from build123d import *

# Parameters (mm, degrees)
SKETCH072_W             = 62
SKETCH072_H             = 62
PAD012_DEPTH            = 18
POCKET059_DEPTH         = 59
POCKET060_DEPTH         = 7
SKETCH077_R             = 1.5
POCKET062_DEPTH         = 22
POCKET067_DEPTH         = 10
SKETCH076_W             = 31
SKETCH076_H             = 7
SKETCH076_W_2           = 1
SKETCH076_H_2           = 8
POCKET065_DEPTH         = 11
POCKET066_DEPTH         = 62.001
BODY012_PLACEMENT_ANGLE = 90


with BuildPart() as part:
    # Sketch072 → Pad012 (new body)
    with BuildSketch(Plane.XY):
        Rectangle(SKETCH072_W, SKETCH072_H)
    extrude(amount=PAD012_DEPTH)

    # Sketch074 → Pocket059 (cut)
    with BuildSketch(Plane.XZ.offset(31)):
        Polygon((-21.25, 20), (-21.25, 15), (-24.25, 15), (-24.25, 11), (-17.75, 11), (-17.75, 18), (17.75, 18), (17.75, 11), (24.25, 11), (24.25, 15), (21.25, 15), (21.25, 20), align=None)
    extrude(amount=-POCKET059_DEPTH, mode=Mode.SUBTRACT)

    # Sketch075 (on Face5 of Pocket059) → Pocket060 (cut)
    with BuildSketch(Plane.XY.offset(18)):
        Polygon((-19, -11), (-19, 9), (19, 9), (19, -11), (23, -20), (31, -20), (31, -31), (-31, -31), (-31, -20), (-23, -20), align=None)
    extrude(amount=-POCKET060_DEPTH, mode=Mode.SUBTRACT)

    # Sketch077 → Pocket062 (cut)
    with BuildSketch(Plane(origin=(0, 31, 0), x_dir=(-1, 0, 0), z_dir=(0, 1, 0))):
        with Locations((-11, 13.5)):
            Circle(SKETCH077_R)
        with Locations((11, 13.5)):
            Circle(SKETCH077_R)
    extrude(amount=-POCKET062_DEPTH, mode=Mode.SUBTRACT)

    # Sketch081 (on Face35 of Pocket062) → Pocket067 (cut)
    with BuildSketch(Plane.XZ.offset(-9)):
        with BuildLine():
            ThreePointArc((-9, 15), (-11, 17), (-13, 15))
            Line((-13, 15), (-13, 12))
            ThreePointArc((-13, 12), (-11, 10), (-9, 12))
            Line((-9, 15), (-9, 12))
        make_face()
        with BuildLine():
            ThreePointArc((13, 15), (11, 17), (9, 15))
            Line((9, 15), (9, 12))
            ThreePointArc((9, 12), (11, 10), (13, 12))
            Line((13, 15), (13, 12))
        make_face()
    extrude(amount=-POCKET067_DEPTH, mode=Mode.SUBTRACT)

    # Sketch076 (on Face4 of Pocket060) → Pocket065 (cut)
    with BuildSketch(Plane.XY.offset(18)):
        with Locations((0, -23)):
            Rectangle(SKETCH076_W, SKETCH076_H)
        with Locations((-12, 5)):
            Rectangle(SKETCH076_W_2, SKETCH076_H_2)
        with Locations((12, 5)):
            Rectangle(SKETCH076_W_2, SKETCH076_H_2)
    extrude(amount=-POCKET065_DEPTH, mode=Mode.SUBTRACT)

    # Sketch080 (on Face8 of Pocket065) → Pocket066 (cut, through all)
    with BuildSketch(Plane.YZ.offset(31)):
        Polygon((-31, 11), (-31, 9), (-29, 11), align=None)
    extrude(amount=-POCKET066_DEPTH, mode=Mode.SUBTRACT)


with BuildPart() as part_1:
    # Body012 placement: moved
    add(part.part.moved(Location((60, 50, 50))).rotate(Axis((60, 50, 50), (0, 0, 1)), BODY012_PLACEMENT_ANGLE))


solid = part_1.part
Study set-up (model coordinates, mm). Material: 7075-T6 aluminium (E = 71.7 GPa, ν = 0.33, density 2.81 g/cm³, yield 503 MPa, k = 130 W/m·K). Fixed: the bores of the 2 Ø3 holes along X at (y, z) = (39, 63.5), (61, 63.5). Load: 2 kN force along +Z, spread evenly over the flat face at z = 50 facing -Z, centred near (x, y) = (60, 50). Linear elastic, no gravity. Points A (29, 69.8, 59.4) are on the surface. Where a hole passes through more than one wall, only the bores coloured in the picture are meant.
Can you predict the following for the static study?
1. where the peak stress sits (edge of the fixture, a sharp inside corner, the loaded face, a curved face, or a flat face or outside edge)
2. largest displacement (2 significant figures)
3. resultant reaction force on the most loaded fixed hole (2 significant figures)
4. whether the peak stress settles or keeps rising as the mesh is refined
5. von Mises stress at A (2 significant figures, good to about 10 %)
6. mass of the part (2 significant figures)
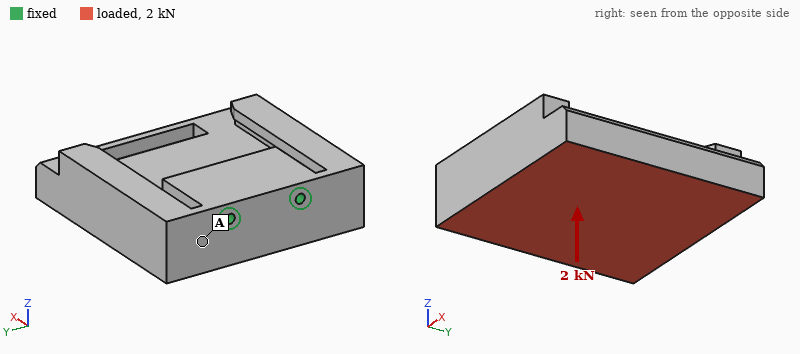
edge of the fixture
92 µm
1.0 kN
keeps rising
15 MPa
150 g
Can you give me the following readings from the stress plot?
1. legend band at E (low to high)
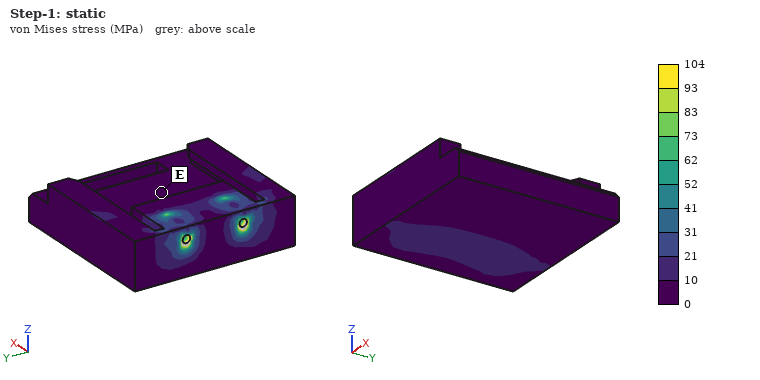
0 to 10 MPa
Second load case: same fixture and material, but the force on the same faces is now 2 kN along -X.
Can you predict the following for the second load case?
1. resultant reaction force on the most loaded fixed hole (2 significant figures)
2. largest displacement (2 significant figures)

1.0 kN
43 µm
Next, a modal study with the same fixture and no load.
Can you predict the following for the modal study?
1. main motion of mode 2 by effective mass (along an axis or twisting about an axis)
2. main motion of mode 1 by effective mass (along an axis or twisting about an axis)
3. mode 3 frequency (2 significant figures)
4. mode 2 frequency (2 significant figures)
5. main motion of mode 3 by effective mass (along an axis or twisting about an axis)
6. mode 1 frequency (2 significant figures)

along Y
along Z
5300 Hz
4500 Hz
along Y
2600 Hz
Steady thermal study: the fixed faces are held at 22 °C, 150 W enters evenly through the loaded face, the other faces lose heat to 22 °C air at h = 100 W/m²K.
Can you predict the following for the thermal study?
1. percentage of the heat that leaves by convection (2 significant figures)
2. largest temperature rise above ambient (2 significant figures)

18 %
43 K
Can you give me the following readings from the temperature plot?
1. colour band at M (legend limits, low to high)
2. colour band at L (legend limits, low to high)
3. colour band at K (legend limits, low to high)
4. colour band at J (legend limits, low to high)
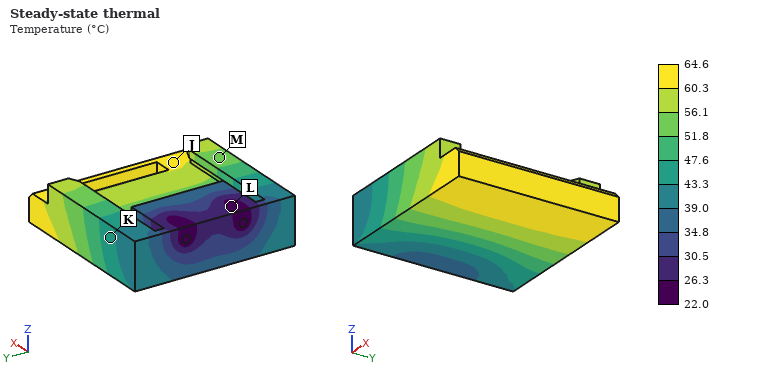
51.8 to 56.1 °C
22.0 to 26.3 °C
43.3 to 47.6 °C
60.3 to 64.6 °C
